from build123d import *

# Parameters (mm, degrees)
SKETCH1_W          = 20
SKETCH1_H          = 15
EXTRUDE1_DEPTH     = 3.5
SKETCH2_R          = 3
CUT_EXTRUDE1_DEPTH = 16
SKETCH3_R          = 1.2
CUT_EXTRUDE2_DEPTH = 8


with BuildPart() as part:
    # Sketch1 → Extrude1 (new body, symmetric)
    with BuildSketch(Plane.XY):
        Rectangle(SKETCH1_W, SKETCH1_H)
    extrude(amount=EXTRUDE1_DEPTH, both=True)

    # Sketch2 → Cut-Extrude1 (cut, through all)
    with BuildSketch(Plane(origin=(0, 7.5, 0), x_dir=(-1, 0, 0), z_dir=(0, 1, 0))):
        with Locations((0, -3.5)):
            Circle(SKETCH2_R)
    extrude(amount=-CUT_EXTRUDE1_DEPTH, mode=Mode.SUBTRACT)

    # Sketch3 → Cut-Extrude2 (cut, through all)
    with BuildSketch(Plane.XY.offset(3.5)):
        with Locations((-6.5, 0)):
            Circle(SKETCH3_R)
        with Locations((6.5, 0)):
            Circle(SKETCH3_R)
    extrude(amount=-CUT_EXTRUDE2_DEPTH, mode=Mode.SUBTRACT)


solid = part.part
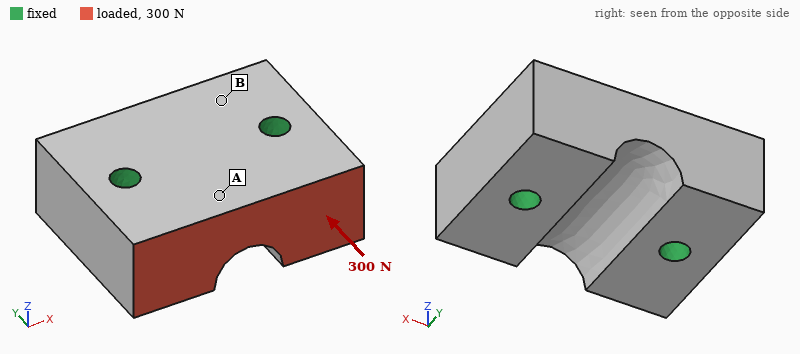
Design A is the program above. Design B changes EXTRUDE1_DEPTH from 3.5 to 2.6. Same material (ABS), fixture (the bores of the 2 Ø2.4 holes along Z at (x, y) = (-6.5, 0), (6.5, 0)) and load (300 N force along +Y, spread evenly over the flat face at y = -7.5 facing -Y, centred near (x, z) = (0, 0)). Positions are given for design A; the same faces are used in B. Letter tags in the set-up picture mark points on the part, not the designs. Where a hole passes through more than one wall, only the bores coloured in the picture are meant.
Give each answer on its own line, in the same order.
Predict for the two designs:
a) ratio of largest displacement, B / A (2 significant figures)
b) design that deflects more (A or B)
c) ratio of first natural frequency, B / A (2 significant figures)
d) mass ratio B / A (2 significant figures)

1.3
B
0.85
0.76
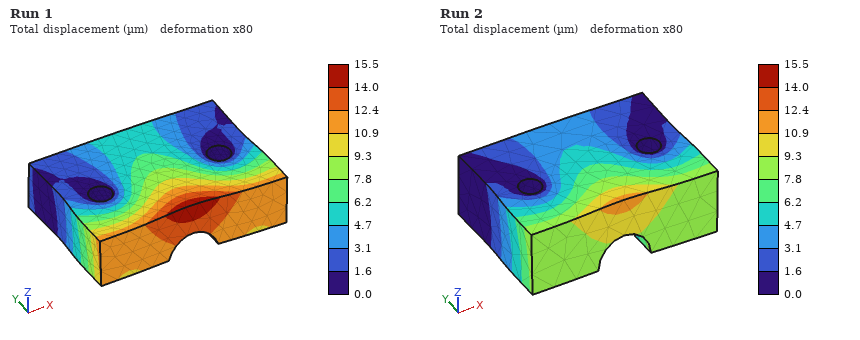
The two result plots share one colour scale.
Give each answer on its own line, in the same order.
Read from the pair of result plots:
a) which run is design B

Run 1
